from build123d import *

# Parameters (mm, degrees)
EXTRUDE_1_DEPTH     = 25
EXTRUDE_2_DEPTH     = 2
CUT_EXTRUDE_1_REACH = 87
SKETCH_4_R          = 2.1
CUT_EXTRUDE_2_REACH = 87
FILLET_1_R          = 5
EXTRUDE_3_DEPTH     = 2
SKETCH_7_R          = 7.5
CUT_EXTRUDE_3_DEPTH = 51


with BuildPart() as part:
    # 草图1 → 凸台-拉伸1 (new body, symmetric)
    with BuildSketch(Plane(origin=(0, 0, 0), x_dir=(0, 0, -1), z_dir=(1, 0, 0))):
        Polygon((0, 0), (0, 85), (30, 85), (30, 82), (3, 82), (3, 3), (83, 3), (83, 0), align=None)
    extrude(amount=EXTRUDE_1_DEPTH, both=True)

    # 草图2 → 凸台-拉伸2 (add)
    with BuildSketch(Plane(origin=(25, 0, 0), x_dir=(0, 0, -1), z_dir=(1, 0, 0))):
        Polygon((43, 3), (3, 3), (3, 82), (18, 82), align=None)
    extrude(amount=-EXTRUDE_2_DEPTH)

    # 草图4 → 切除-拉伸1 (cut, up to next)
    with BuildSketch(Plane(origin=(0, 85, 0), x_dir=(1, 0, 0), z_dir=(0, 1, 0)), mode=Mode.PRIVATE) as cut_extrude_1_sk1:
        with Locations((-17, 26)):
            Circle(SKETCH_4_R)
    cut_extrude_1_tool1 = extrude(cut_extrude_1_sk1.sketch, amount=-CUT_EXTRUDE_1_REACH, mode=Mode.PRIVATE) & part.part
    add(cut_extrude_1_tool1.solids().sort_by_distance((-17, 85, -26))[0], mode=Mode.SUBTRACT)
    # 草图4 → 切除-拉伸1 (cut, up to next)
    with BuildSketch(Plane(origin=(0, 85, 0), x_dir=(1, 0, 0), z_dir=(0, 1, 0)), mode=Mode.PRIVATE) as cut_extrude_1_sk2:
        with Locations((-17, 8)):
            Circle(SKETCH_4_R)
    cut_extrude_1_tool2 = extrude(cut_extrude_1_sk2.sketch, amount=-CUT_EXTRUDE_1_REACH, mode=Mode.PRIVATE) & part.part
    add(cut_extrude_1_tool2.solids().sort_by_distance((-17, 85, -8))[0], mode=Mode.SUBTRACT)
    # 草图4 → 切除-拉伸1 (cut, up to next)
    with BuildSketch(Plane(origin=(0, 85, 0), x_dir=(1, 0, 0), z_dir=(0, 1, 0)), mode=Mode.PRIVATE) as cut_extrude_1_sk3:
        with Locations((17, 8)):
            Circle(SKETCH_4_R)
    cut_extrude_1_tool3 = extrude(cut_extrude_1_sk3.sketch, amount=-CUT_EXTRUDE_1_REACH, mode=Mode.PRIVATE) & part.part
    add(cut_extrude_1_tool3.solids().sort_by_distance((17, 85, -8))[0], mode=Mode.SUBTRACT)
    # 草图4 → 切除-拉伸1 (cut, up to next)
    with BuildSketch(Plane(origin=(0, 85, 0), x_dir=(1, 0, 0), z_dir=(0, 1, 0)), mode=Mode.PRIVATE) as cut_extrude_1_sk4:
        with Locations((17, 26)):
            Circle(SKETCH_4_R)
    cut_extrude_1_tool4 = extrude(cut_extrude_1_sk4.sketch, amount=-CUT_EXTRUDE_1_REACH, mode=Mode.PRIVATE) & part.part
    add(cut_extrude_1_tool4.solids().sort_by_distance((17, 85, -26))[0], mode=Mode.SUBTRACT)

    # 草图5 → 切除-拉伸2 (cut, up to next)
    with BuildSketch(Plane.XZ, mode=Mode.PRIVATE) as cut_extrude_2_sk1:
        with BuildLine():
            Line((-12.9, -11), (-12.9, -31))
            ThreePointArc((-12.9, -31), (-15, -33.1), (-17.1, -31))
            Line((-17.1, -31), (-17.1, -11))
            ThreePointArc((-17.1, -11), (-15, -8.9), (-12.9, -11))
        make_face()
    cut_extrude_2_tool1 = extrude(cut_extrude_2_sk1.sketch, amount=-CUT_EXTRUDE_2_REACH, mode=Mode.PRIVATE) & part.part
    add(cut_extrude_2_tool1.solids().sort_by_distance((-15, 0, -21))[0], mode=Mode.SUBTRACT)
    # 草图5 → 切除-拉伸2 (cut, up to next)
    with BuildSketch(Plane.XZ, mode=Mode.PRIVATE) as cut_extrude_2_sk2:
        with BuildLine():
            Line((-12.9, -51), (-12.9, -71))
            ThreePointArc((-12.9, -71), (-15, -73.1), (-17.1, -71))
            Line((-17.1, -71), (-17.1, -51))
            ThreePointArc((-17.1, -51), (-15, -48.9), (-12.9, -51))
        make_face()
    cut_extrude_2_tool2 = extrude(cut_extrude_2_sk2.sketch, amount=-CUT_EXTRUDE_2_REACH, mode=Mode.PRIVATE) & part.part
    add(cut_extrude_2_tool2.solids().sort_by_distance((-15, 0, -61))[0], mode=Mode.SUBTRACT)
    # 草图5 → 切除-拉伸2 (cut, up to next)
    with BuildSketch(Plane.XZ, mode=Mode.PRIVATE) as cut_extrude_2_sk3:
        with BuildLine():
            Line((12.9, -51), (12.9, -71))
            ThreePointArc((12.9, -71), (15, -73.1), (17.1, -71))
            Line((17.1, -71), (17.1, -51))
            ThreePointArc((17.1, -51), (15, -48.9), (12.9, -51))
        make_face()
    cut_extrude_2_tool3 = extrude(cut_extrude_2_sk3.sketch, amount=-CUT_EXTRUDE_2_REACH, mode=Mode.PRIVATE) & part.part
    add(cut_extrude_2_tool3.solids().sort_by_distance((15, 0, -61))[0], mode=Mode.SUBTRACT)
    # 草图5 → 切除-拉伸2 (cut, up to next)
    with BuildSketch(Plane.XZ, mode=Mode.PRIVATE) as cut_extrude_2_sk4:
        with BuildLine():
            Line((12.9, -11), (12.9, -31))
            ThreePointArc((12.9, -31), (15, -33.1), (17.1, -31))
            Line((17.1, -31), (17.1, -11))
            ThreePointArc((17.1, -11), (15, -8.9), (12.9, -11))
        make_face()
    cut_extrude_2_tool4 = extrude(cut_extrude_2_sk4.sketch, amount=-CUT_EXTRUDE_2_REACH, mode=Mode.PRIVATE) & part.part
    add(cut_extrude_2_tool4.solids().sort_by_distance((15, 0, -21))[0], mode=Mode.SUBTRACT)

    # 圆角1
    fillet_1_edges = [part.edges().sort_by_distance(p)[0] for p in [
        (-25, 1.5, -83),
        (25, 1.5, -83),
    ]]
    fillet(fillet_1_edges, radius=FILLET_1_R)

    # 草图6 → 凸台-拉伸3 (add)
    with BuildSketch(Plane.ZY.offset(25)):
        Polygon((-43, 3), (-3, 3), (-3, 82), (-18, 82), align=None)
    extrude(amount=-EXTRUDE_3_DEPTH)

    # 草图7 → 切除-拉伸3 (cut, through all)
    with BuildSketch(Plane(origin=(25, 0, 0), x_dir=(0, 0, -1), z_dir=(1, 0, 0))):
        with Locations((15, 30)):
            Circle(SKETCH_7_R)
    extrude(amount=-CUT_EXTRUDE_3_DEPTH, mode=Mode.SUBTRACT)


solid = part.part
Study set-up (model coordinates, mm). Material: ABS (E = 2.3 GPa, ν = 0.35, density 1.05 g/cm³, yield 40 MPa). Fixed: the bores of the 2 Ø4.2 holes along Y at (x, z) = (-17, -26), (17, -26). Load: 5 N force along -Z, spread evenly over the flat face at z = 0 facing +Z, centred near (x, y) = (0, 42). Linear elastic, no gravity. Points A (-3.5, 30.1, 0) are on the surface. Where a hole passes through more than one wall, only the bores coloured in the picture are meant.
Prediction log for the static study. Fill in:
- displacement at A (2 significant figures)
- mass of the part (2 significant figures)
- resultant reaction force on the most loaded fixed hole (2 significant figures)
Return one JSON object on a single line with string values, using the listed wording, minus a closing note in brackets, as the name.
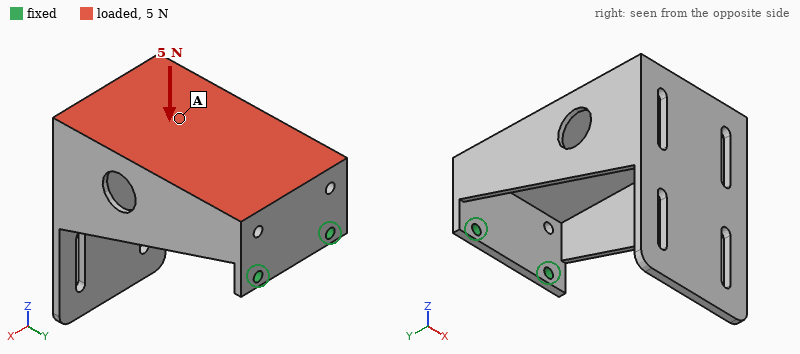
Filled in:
{"displacement at A": "0.70 mm", "mass of the part": "37 g", "resultant reaction force on the most loaded fixed hole": "2.6 N"}
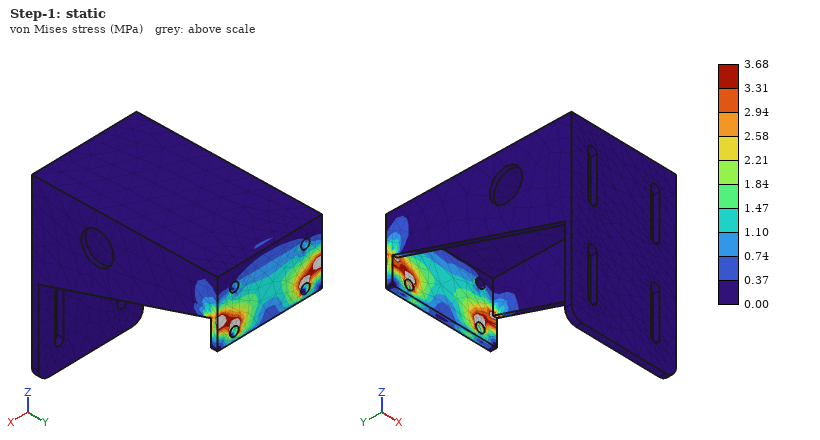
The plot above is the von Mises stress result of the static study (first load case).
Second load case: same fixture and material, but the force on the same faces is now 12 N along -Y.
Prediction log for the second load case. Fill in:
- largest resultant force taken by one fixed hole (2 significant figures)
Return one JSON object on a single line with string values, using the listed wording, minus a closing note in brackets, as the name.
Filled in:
{"largest resultant force taken by one fixed hole": "6.0 N"}
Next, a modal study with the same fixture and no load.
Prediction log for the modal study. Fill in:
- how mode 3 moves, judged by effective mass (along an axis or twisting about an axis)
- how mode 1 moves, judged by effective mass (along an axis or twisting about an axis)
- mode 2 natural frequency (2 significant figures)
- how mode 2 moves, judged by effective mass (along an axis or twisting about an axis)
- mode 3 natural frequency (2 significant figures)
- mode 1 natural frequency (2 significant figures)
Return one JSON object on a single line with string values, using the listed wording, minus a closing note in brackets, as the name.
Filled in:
{"how mode 3 moves, judged by effective mass": "along Y", "how mode 1 moves, judged by effective mass": "along Z", "mode 2 natural frequency": "72 Hz", "how mode 2 moves, judged by effective mass": "along X", "mode 3 natural frequency": "290 Hz", "mode 1 natural frequency": "53 Hz"}
